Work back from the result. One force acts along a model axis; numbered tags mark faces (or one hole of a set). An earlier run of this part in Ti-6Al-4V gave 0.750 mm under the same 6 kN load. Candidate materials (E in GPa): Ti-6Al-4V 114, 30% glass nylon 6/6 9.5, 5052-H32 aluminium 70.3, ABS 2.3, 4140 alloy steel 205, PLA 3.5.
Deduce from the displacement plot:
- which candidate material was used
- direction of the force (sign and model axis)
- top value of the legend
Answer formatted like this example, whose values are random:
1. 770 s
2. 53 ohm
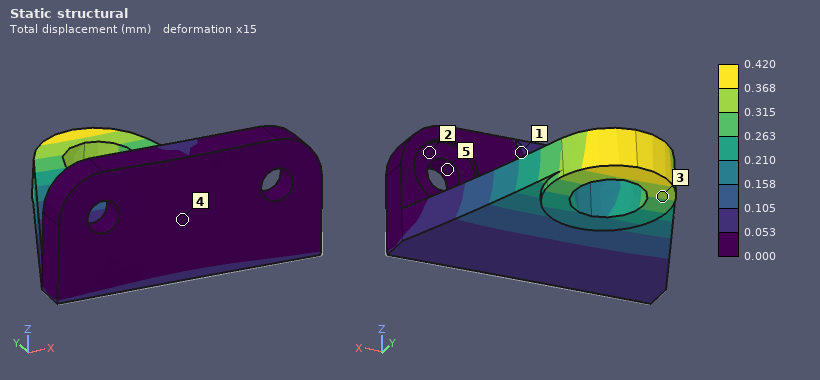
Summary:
1. 4140 alloy steel
2. +Z
3. 0.420 mm
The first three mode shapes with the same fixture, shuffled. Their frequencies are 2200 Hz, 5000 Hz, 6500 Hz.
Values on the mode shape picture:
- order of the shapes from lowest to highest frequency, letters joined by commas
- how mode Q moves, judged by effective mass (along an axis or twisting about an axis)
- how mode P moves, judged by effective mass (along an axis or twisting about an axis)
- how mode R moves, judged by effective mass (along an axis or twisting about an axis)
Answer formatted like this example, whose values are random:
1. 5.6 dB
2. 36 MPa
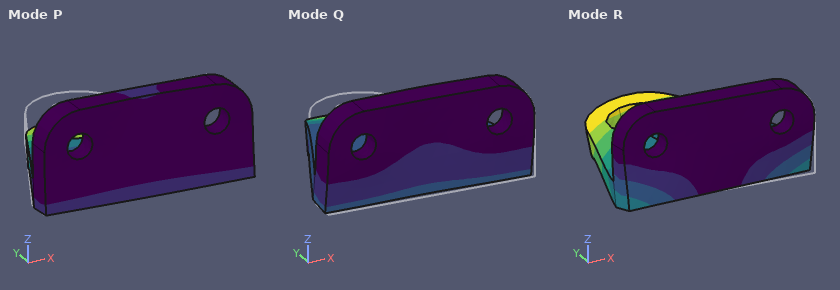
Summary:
1. P, R, Q
2. along Y
3. along Z
4. along X
